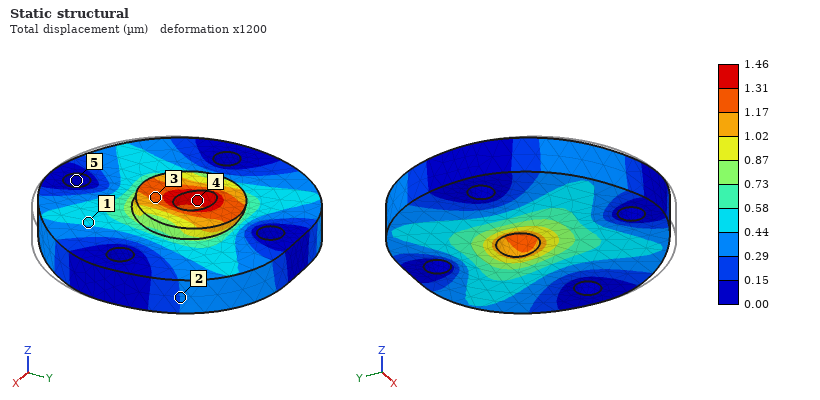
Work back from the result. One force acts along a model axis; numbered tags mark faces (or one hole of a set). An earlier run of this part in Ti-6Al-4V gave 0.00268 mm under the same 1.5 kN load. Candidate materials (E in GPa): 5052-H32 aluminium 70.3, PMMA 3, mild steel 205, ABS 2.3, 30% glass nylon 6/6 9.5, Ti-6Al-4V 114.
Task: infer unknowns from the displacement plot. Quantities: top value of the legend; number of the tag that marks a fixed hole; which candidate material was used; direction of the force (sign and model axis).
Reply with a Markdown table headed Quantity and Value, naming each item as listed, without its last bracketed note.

| Quantity | Value |
|---|---|
| top value of the legend | 1.46 µm |
| number of the tag that marks a fixed hole | 5 |
| which candidate material was used | mild steel |
| direction of the force | +Y |
